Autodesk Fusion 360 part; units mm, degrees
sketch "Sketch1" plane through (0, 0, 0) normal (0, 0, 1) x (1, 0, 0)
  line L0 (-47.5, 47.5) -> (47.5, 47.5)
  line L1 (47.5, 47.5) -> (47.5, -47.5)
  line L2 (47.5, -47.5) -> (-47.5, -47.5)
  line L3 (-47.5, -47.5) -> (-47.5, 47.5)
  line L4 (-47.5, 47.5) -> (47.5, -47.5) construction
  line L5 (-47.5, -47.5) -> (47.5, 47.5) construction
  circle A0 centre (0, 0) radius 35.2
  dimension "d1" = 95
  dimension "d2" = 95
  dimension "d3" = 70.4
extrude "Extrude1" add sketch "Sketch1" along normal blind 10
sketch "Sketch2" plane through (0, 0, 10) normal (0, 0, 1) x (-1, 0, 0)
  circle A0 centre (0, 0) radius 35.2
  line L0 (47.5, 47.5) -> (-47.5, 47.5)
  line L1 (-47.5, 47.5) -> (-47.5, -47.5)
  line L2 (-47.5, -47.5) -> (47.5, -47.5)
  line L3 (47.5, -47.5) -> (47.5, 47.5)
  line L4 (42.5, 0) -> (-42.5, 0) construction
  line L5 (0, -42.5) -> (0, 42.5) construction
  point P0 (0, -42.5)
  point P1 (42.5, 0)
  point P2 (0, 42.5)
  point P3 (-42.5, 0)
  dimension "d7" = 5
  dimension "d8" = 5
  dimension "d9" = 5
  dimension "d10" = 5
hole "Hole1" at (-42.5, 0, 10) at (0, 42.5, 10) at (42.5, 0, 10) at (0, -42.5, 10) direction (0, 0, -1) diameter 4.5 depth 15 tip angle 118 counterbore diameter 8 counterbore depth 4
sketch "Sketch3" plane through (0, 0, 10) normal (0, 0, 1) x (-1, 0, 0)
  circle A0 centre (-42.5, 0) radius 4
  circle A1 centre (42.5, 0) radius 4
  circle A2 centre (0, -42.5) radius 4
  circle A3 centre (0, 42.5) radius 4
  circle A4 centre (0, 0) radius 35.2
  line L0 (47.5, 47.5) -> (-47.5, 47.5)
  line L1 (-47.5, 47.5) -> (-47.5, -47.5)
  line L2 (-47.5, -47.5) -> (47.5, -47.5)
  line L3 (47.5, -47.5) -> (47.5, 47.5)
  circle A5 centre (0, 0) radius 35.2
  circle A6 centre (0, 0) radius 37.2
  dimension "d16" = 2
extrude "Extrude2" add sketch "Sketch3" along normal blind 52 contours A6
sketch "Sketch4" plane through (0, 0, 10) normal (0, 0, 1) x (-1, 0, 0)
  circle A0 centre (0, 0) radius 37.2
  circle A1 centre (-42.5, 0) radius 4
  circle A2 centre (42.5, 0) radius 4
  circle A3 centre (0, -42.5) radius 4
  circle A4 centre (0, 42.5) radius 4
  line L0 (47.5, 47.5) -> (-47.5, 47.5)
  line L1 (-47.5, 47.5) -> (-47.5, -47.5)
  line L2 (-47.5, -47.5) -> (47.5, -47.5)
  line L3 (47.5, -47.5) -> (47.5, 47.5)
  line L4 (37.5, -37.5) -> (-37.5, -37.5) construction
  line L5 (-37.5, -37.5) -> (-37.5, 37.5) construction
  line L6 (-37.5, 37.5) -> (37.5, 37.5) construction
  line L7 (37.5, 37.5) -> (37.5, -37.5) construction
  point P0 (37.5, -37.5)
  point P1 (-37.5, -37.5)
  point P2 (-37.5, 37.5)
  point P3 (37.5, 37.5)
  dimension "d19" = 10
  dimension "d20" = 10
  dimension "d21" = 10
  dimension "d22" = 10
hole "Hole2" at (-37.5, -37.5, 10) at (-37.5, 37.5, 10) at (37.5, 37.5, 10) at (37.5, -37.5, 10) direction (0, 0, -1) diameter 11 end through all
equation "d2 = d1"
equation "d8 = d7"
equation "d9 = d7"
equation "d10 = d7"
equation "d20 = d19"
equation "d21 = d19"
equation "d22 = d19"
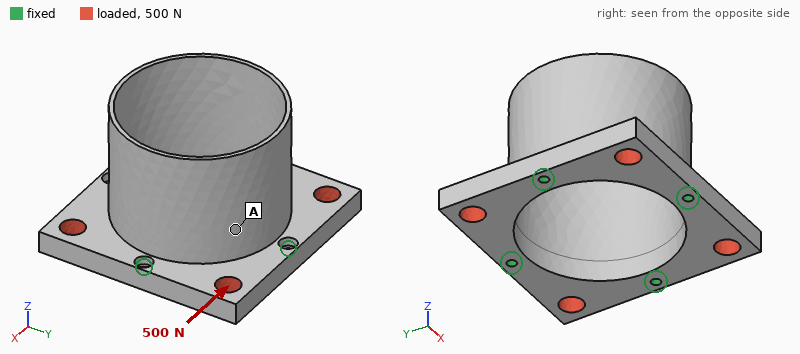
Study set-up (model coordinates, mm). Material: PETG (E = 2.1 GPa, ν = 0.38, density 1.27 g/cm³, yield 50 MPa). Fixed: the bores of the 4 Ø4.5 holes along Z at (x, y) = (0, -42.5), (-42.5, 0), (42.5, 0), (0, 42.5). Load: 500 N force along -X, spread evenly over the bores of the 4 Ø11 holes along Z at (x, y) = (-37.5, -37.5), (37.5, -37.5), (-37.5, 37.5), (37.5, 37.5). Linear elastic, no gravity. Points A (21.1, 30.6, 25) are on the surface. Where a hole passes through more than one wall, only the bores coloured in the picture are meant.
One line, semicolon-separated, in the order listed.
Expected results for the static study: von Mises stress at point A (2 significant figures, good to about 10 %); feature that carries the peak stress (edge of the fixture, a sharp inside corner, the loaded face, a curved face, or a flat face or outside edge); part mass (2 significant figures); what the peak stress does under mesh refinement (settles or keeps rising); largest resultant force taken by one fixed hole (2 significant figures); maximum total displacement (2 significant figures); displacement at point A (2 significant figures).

0.17 MPa; edge of the fixture; 89 g; keeps rising; 230 N; 26 µm; 19 µm
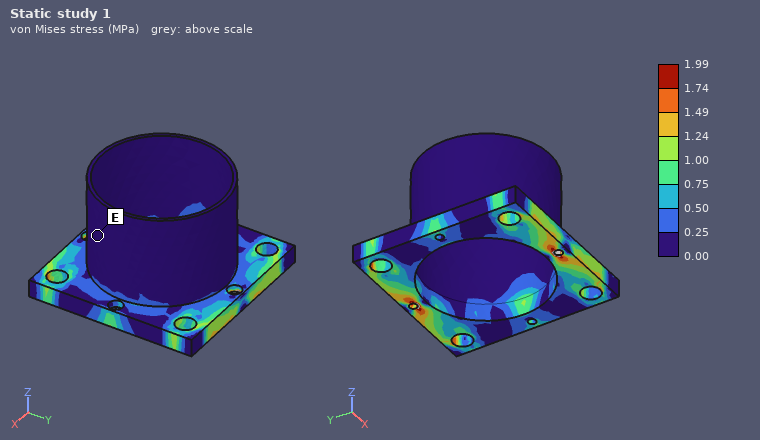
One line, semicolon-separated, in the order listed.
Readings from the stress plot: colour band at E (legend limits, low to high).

0.00 to 0.25 MPa
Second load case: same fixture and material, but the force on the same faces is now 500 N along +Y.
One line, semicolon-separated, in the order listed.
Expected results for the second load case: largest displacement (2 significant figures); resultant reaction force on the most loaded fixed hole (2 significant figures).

26 µm; 230 N
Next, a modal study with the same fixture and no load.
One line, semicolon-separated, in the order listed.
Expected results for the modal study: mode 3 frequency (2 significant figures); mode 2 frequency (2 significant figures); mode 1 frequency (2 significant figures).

920 Hz; 920 Hz; 640 Hz
